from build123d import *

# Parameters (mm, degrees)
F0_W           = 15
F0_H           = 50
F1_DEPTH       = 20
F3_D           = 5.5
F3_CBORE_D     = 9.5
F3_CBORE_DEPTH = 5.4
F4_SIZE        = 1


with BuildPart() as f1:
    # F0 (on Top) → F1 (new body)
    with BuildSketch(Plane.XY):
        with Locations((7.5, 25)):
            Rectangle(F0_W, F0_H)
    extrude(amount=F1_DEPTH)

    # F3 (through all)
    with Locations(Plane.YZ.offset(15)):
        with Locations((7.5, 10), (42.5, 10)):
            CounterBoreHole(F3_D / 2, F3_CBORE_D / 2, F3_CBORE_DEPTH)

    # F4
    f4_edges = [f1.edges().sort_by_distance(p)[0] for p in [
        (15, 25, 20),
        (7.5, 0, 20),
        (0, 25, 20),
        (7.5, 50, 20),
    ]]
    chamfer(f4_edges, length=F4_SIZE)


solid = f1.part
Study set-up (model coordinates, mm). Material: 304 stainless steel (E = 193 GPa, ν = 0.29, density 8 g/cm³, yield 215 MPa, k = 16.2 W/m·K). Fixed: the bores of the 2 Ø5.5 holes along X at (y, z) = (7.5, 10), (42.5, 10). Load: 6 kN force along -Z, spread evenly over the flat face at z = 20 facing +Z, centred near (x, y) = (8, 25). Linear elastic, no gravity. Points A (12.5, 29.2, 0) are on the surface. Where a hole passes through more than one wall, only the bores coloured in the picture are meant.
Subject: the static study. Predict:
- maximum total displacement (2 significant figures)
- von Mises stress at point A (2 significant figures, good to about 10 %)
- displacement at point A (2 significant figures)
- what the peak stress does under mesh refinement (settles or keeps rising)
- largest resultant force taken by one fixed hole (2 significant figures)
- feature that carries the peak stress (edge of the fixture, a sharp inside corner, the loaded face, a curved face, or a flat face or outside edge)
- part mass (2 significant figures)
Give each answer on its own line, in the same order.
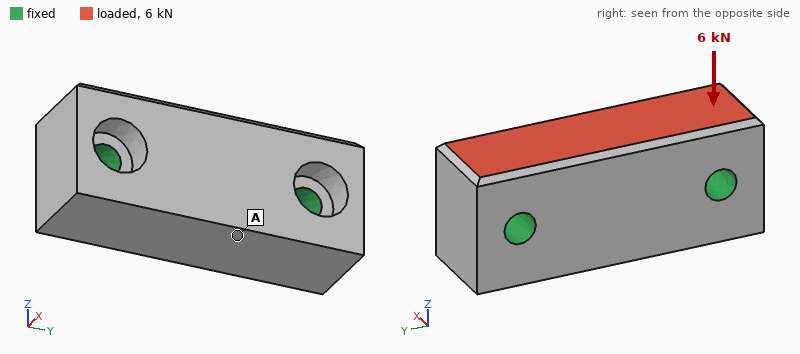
3.1 µm
11 MPa
2.5 µm
keeps rising
3.0 kN
edge of the fixture
110 g
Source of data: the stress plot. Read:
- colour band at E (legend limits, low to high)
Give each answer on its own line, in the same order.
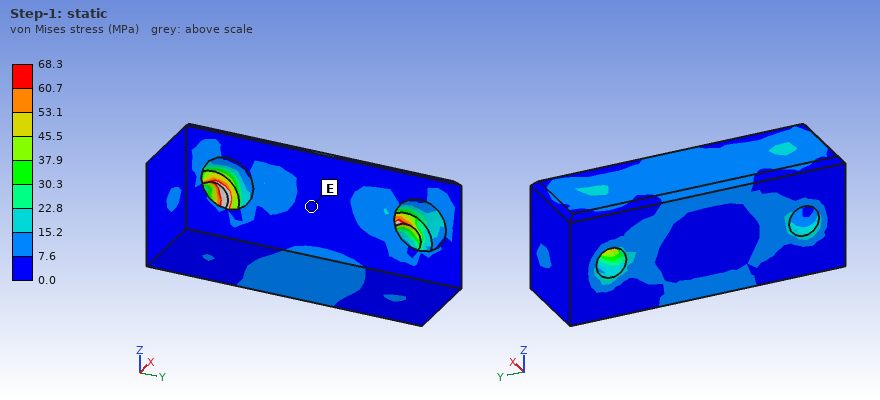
0.0 to 7.6 MPa
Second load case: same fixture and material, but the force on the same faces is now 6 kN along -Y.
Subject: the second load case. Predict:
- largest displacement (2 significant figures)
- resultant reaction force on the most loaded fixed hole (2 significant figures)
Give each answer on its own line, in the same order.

2.6 µm
3.3 kN
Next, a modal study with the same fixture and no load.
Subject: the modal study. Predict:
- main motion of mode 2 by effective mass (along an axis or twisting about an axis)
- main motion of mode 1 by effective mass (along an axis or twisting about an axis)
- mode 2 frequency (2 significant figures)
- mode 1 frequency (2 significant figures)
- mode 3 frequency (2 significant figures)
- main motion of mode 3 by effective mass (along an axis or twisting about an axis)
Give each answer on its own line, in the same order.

along X
along Z
28 kHz
24 kHz
31 kHz
along Z
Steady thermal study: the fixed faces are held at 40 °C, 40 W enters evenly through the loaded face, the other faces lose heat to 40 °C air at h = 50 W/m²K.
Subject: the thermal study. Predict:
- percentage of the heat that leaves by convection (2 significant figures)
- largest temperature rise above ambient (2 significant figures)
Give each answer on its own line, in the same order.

9.4 %
60 K
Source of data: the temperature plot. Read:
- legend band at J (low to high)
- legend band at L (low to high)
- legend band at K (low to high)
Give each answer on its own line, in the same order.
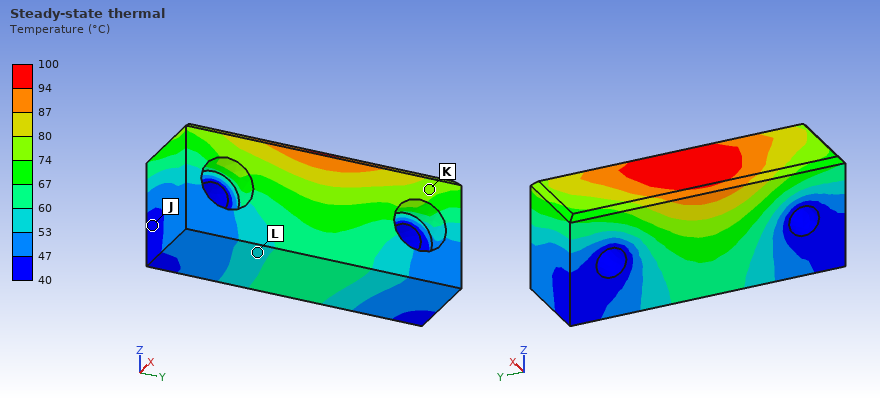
40 to 47 °C
53 to 60 °C
74 to 80 °C
